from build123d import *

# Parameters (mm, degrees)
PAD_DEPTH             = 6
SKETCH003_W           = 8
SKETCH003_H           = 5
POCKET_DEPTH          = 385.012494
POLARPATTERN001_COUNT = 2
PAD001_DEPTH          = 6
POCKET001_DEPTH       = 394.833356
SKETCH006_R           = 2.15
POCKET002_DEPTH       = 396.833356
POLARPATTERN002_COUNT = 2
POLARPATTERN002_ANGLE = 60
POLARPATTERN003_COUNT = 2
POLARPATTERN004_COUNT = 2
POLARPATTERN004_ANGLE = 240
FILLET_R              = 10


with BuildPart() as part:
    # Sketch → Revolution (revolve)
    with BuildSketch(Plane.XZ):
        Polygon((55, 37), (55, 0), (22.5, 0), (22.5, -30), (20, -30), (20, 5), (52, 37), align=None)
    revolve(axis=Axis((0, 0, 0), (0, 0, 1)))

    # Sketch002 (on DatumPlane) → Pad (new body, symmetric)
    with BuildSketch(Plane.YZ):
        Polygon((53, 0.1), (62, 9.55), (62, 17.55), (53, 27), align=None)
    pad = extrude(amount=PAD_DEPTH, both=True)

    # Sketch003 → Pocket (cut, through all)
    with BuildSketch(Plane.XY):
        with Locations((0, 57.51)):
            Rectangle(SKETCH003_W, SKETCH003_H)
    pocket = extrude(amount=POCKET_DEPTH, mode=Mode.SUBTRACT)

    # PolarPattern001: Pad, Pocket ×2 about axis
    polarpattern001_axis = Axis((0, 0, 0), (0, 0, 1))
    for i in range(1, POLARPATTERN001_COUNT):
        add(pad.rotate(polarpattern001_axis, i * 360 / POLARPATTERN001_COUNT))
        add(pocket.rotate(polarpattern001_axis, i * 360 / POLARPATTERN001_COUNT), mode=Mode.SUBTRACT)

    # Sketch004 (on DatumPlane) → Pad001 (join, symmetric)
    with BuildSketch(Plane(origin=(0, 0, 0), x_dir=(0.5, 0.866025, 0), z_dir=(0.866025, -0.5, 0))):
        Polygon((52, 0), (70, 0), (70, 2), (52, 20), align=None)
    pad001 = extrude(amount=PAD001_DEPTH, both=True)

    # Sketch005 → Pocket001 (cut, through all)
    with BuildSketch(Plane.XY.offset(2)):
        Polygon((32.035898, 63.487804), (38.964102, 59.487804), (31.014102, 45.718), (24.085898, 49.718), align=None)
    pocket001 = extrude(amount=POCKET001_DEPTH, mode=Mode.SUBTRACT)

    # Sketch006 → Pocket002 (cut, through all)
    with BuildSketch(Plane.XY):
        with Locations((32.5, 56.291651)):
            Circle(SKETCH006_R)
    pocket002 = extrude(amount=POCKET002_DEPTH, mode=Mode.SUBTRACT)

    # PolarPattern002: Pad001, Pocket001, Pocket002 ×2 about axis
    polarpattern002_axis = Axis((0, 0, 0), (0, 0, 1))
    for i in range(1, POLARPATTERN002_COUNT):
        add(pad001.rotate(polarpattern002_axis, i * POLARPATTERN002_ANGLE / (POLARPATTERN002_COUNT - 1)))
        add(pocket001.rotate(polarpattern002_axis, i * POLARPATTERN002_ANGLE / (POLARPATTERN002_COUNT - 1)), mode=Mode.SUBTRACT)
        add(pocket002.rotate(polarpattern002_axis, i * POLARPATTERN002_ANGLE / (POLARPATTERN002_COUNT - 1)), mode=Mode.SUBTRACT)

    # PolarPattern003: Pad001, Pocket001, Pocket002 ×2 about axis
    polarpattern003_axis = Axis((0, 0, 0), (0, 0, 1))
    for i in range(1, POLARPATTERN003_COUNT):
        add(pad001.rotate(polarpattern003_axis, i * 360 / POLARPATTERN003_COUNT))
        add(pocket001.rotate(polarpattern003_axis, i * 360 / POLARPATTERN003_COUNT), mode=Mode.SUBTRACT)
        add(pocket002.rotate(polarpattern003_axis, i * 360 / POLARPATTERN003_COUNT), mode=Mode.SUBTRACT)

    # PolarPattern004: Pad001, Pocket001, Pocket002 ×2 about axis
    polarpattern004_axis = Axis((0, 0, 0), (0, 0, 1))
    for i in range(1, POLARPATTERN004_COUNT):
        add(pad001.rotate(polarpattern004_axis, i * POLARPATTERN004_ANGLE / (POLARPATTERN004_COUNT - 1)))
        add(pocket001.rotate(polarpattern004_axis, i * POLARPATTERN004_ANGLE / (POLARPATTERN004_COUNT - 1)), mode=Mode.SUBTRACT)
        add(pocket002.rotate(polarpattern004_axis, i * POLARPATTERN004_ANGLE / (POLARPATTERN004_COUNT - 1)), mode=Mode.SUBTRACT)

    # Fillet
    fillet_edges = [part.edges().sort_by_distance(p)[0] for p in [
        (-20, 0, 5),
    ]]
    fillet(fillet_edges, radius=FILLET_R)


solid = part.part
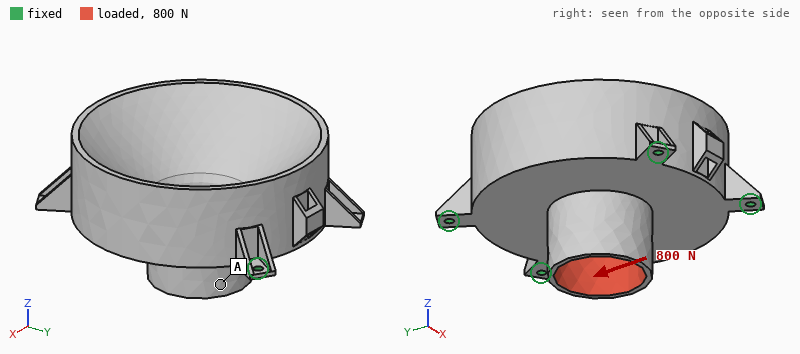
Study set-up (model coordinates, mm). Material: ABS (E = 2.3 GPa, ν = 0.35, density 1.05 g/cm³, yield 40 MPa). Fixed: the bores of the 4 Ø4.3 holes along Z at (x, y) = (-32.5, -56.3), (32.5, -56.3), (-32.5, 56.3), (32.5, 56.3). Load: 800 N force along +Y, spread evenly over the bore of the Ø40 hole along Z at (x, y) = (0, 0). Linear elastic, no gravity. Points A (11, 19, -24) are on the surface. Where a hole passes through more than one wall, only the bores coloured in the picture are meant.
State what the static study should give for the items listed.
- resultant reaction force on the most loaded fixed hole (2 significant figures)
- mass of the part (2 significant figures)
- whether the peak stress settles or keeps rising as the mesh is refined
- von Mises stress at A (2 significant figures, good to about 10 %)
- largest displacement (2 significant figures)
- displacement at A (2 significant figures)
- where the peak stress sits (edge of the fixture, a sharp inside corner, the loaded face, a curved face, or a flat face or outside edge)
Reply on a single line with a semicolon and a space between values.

220 N; 230 g; keeps rising; 1.7 MPa; 0.31 mm; 0.27 mm; edge of the fixture
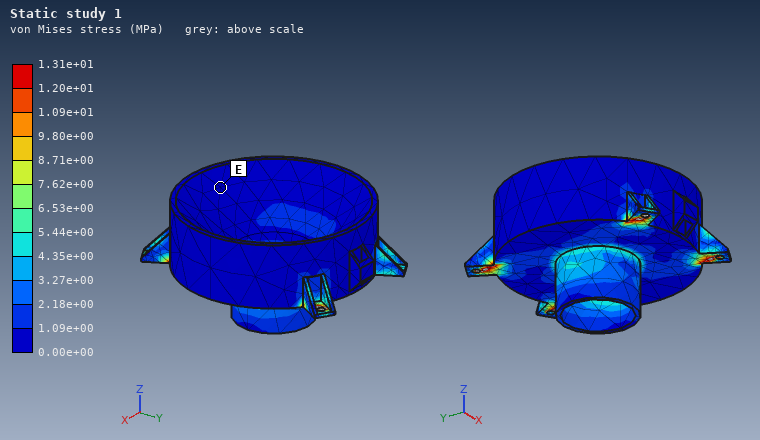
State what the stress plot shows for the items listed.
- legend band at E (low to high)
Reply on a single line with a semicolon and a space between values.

0.00e+00 to 1.09e+00 MPa
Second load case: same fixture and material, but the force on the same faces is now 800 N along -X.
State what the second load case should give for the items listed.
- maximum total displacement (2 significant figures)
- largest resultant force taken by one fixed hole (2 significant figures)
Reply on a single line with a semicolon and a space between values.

0.43 mm; 230 N
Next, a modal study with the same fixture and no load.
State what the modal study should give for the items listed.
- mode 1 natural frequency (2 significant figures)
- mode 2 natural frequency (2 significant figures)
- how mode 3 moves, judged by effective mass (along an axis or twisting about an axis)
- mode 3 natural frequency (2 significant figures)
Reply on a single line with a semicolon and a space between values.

670 Hz; 690 Hz; along X; 980 Hz
